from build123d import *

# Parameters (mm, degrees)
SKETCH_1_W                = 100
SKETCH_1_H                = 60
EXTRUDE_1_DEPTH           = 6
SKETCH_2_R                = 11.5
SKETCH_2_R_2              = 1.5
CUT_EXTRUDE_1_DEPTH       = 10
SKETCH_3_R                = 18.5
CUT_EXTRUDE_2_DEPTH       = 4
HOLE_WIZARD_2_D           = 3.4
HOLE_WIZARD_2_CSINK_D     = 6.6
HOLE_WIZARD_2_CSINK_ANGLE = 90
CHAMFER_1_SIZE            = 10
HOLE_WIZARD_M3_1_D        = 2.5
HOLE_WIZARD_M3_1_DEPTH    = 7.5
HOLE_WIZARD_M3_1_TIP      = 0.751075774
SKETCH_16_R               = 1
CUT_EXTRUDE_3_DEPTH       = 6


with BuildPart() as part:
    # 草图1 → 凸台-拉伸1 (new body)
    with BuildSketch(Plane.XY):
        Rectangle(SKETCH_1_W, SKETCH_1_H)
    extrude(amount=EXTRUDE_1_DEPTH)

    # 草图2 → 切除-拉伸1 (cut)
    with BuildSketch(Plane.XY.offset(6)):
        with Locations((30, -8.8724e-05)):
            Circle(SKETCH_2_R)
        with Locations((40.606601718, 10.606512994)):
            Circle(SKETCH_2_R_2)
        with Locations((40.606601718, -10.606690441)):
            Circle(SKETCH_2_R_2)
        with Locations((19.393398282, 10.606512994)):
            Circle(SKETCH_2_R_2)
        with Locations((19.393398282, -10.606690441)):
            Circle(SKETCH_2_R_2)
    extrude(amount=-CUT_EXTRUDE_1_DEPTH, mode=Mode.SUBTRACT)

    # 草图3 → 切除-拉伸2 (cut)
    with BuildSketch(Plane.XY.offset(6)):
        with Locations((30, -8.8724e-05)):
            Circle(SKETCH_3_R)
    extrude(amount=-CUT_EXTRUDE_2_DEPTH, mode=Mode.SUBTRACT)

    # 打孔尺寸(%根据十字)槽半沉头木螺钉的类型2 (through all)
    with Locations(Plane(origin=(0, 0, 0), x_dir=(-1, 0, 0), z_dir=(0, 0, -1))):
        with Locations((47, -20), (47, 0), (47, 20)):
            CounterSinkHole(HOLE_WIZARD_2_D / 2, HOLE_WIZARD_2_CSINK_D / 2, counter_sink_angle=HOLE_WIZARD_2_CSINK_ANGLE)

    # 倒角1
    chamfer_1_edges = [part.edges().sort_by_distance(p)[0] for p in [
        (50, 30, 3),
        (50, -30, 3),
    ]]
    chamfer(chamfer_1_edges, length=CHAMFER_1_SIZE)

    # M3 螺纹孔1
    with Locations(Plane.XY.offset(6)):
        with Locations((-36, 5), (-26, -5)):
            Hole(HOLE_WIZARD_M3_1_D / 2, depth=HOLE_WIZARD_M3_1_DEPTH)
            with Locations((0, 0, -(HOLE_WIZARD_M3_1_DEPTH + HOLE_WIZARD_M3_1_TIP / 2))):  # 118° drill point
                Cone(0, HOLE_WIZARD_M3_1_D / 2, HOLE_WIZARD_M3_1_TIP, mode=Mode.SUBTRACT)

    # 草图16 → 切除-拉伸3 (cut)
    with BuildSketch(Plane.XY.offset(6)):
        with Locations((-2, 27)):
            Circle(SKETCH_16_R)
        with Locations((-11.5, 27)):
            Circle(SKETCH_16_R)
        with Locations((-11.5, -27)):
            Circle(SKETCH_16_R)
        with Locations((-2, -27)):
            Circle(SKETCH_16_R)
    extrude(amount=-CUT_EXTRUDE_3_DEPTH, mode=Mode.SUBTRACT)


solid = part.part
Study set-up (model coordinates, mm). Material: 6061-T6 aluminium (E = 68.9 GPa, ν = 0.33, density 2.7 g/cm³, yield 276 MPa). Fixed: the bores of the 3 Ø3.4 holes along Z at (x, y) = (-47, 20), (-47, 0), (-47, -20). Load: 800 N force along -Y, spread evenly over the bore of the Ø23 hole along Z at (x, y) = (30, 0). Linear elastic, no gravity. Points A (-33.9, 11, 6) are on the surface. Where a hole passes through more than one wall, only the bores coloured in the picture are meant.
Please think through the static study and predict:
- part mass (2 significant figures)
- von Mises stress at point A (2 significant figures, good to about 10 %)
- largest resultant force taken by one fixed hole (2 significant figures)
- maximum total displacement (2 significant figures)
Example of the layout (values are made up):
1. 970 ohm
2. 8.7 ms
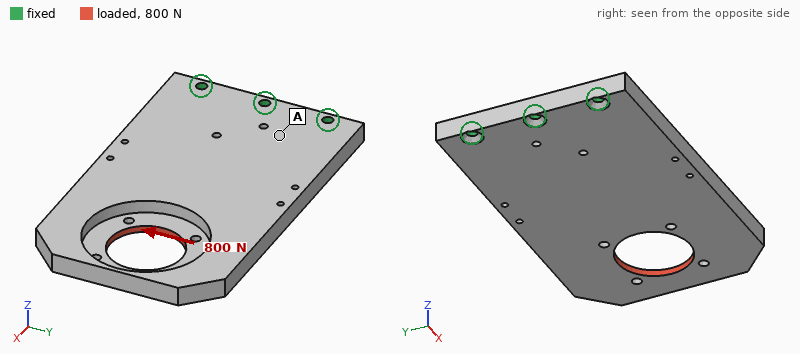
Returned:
1. 81 g
2. 8.5 MPa
3. 1.5 kN
4. 56 µm
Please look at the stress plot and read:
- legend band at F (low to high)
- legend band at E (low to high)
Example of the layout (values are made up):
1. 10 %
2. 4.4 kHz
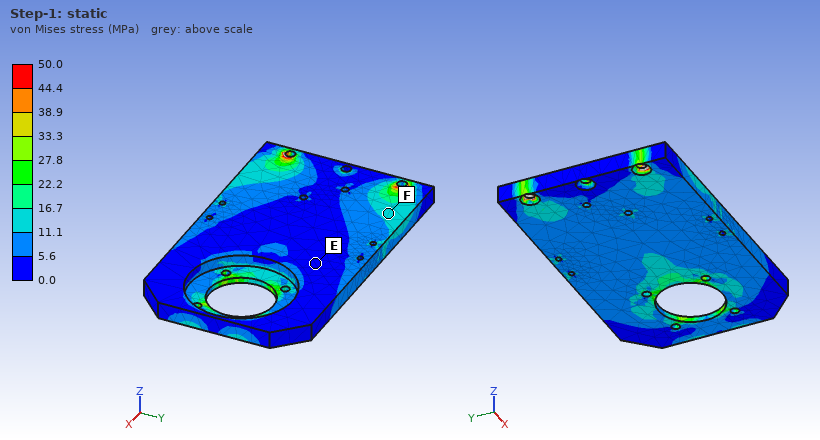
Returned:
1. 11.1 to 16.7 MPa
2. 0.0 to 5.6 MPa
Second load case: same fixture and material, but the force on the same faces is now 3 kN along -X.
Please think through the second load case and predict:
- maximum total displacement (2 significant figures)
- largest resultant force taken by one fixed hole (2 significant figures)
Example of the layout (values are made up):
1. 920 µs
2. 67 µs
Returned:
1. 0.42 mm
2. 1.0 kN
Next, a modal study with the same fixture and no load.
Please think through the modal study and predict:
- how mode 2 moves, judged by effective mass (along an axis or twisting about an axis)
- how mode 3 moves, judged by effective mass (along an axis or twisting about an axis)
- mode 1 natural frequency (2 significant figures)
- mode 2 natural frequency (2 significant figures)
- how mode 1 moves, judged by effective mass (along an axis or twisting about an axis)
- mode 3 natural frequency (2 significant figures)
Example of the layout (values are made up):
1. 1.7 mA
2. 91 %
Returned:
1. twisting about X
2. along Z
3. 600 Hz
4. 1800 Hz
5. along Z
6. 2900 Hz
